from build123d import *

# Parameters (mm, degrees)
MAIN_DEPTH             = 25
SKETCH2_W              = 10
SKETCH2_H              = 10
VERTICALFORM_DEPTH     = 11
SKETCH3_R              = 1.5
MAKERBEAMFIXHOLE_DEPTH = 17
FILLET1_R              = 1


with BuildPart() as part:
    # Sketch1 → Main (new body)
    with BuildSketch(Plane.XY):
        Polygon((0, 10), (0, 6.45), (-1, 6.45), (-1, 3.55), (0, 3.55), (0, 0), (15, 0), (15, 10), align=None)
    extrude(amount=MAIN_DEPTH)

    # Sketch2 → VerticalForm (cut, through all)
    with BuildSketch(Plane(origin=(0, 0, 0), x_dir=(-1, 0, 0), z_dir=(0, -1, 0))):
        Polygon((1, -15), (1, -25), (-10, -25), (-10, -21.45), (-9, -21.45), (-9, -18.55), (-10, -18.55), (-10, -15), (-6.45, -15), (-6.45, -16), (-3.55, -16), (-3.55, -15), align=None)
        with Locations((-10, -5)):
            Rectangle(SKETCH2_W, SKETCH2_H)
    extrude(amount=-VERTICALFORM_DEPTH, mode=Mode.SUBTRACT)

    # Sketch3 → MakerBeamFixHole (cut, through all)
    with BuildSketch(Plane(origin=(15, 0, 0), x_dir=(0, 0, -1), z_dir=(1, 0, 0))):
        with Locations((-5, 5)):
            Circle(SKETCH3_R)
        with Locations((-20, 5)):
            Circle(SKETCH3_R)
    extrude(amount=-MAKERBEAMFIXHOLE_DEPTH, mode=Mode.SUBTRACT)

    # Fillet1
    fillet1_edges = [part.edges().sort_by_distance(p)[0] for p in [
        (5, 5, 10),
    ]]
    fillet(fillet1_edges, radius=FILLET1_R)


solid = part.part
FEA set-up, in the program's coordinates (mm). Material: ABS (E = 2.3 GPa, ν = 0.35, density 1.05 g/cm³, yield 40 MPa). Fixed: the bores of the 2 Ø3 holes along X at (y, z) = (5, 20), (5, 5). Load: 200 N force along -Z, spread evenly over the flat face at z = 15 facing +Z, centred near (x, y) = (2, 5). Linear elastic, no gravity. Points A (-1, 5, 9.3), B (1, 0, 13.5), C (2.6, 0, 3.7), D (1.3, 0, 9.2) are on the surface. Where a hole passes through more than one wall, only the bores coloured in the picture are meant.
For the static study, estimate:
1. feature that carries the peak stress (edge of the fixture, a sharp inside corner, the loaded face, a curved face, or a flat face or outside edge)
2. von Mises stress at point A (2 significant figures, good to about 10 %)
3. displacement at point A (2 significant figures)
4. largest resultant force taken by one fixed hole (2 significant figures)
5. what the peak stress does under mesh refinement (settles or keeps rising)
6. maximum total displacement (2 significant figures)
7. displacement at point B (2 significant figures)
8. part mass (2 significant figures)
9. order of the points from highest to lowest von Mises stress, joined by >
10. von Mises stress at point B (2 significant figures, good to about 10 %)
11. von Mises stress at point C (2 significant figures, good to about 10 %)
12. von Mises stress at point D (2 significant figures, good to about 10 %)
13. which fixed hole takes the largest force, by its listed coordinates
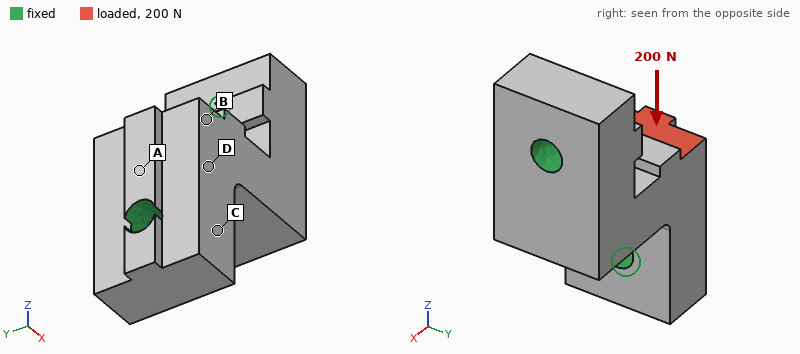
edge of the fixture
6.7 MPa
9.0 µm
200 N
keeps rising
26 µm
19 µm
1.9 g
A > B > D > C
5.1 MPa
1.2 MPa
3.2 MPa
(5, 5)
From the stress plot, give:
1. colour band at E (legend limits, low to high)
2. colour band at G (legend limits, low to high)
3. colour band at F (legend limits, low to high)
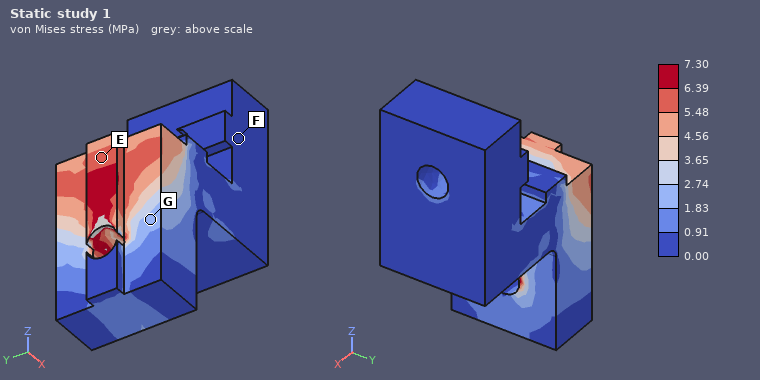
5.48 to 6.39 MPa
1.83 to 2.74 MPa
0.00 to 0.91 MPa
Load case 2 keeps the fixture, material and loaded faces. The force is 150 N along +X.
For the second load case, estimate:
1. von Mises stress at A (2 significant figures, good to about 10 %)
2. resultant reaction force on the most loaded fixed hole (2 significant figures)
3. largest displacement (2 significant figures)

6.3 MPa
80 N
67 µm
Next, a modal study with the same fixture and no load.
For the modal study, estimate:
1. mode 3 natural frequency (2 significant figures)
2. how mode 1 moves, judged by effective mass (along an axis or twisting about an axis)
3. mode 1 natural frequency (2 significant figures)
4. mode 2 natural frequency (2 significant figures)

12 kHz
along Y
11 kHz
12 kHz
